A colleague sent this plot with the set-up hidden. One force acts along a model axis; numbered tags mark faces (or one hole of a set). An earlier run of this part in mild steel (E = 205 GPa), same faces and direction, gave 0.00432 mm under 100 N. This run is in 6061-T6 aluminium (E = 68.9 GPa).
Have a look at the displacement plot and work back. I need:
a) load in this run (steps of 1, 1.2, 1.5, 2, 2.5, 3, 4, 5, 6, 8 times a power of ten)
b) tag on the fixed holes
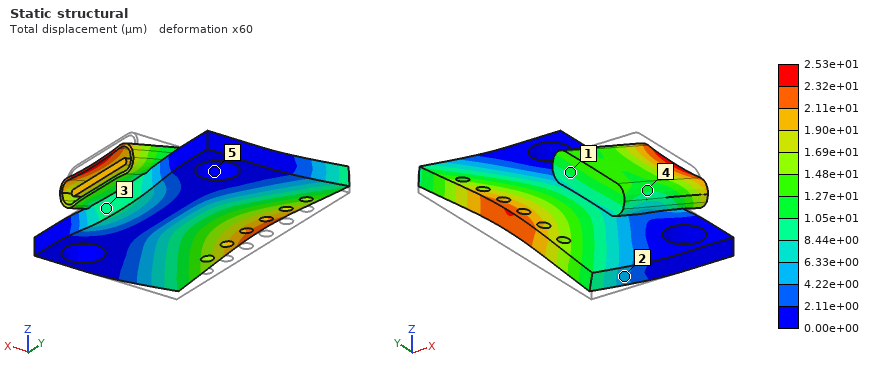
200 N
5
